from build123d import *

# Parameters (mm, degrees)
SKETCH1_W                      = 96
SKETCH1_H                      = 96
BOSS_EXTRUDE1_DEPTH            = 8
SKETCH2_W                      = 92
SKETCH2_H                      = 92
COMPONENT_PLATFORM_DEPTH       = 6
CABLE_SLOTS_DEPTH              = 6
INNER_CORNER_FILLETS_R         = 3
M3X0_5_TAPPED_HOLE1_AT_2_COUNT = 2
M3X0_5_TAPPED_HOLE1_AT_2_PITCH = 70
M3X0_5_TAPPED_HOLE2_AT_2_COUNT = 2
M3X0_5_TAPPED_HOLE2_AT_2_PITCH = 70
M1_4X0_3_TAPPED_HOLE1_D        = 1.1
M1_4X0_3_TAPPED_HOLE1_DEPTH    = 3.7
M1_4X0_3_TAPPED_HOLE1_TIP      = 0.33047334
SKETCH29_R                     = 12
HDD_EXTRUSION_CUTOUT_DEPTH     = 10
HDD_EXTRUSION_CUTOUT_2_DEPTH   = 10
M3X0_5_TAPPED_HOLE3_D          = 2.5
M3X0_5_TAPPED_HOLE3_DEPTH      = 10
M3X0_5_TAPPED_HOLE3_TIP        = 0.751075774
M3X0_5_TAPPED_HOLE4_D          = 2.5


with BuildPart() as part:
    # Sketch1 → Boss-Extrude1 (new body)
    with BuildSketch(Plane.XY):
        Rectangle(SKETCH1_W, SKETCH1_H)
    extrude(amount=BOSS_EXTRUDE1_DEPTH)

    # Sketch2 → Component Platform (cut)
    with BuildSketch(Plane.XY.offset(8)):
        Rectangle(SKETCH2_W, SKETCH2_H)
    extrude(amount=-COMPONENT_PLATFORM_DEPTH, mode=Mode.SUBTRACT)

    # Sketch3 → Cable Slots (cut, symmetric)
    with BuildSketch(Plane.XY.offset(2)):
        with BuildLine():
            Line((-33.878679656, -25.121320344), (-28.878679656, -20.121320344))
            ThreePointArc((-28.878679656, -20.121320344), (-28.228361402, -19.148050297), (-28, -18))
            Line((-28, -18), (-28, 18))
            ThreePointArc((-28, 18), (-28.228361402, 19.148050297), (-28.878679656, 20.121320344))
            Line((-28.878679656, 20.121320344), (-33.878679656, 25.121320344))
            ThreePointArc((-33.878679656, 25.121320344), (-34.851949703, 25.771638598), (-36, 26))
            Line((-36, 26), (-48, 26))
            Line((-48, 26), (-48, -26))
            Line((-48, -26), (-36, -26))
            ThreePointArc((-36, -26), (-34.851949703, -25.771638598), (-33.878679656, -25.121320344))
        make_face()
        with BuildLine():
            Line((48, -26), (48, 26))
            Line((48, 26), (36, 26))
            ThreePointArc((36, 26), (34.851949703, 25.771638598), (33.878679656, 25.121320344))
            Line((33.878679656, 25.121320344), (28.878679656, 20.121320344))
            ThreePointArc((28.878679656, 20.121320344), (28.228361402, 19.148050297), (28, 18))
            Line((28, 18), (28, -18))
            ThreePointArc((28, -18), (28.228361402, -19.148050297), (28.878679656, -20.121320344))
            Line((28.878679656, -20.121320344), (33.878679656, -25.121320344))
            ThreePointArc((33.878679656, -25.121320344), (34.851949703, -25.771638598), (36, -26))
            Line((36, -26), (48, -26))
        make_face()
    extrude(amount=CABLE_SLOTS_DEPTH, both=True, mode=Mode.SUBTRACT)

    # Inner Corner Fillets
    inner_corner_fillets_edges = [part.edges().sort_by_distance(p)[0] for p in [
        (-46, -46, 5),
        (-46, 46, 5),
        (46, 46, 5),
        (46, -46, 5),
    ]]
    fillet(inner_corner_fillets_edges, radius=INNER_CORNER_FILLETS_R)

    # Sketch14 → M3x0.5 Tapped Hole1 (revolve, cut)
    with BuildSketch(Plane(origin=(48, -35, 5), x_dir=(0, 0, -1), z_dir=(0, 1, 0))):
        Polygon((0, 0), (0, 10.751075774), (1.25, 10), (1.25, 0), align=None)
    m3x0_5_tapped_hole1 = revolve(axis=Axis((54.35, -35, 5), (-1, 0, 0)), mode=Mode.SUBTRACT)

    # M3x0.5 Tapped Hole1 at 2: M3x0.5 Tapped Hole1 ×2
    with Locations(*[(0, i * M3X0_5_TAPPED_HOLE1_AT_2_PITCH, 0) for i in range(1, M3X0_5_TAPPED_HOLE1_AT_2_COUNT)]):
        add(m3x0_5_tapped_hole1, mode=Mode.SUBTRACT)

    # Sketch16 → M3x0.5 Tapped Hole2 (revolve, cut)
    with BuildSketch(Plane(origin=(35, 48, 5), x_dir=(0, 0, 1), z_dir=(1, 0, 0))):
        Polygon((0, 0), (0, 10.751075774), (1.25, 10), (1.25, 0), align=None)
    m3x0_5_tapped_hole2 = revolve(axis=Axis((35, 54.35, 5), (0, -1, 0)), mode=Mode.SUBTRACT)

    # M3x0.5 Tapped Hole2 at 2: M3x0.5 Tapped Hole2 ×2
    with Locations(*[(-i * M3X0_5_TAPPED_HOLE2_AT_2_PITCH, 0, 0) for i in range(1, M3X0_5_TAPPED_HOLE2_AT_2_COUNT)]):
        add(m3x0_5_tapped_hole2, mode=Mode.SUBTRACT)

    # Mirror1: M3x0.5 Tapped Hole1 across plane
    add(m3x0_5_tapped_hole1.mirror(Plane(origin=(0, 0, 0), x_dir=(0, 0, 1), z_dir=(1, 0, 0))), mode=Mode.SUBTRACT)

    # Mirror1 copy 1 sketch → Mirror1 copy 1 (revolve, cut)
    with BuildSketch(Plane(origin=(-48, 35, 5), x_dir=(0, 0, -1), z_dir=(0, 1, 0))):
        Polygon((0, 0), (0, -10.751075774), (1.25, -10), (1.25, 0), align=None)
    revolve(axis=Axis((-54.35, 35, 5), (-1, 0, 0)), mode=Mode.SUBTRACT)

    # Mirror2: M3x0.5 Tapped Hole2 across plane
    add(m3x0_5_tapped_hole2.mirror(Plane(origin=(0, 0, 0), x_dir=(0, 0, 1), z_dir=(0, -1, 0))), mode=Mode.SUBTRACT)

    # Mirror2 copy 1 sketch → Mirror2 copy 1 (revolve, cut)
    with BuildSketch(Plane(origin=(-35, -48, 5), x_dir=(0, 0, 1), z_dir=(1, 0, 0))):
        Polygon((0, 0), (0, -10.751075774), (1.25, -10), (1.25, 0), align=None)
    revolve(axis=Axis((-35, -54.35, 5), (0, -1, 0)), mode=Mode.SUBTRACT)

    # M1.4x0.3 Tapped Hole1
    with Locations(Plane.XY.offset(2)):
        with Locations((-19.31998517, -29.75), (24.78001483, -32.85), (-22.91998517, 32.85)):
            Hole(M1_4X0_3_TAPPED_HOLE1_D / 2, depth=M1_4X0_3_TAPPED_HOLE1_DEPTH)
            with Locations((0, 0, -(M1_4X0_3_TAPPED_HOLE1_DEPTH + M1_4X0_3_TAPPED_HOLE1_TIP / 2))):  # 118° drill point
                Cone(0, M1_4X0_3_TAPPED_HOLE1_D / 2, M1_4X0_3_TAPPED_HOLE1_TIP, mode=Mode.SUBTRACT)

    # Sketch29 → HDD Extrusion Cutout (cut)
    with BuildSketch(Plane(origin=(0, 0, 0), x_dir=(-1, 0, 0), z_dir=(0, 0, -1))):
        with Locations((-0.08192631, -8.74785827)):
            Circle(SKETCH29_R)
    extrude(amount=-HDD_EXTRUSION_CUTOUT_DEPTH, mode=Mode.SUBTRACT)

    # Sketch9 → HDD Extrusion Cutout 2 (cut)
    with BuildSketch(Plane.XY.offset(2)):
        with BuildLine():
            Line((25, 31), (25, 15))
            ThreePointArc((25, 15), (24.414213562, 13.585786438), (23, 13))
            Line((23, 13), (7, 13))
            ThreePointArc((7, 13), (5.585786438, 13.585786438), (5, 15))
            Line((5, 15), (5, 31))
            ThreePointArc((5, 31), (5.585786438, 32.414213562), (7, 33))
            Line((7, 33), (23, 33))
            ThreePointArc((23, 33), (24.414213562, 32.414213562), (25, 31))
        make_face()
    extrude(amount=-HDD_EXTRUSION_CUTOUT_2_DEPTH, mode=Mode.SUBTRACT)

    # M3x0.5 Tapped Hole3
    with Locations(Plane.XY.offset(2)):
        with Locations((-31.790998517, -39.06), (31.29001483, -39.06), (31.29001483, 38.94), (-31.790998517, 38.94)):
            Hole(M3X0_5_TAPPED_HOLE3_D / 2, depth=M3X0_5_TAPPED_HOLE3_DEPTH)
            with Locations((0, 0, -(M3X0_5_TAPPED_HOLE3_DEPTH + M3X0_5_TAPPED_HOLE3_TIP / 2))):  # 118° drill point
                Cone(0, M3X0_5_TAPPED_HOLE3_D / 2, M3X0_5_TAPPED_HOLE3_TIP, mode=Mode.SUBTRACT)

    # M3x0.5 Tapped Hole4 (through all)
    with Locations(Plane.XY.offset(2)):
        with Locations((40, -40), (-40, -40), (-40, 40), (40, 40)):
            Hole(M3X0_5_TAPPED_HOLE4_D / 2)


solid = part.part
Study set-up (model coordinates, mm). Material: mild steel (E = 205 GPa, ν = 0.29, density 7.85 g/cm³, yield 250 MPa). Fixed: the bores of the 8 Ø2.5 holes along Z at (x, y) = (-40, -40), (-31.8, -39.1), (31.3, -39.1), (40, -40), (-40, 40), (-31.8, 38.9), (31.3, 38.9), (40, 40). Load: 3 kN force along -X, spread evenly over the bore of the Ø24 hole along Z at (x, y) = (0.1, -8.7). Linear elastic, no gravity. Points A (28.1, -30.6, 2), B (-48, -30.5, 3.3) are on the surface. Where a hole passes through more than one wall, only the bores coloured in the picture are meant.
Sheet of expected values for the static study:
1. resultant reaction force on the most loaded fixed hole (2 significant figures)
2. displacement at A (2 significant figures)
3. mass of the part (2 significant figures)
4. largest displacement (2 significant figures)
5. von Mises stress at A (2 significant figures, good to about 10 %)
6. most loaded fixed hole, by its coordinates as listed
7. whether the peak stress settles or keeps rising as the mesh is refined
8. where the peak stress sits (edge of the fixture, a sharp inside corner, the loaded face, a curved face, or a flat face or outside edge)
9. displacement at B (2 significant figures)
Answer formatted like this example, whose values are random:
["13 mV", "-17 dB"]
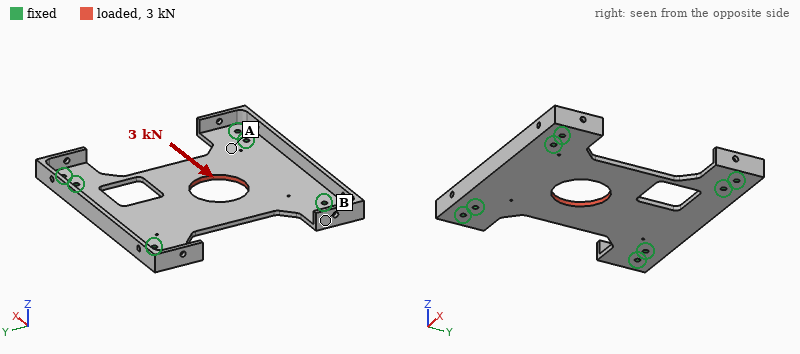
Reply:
["770 N", "1.9 µm", "120 g", "11 µm", "21 MPa", "(-31.8, -39.1)", "keeps rising", "a sharp inside corner", "2.1 µm"]
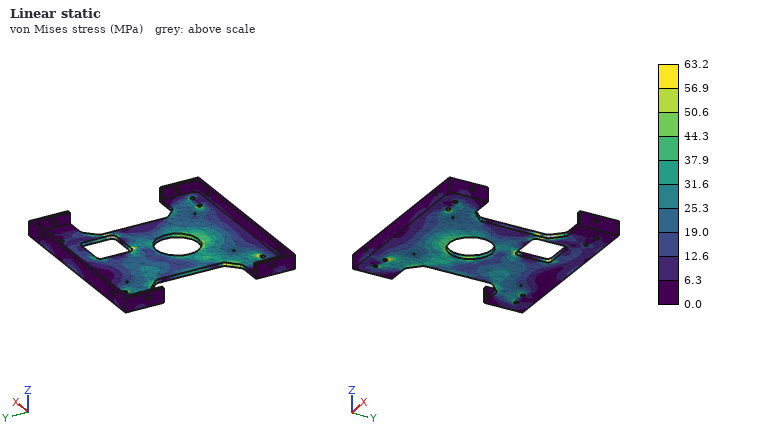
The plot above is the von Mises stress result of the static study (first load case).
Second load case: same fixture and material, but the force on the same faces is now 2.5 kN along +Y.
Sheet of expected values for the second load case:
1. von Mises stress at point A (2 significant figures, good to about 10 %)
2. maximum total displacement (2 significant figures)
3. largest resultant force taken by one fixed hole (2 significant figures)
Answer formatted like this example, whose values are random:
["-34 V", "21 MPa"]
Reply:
["28 MPa", "8.3 µm", "820 N"]
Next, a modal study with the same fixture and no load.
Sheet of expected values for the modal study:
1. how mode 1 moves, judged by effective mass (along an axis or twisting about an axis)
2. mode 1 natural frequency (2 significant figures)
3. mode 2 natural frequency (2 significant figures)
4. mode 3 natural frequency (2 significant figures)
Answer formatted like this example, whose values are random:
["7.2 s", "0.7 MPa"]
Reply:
["along Z", "1400 Hz", "2500 Hz", "3200 Hz"]
